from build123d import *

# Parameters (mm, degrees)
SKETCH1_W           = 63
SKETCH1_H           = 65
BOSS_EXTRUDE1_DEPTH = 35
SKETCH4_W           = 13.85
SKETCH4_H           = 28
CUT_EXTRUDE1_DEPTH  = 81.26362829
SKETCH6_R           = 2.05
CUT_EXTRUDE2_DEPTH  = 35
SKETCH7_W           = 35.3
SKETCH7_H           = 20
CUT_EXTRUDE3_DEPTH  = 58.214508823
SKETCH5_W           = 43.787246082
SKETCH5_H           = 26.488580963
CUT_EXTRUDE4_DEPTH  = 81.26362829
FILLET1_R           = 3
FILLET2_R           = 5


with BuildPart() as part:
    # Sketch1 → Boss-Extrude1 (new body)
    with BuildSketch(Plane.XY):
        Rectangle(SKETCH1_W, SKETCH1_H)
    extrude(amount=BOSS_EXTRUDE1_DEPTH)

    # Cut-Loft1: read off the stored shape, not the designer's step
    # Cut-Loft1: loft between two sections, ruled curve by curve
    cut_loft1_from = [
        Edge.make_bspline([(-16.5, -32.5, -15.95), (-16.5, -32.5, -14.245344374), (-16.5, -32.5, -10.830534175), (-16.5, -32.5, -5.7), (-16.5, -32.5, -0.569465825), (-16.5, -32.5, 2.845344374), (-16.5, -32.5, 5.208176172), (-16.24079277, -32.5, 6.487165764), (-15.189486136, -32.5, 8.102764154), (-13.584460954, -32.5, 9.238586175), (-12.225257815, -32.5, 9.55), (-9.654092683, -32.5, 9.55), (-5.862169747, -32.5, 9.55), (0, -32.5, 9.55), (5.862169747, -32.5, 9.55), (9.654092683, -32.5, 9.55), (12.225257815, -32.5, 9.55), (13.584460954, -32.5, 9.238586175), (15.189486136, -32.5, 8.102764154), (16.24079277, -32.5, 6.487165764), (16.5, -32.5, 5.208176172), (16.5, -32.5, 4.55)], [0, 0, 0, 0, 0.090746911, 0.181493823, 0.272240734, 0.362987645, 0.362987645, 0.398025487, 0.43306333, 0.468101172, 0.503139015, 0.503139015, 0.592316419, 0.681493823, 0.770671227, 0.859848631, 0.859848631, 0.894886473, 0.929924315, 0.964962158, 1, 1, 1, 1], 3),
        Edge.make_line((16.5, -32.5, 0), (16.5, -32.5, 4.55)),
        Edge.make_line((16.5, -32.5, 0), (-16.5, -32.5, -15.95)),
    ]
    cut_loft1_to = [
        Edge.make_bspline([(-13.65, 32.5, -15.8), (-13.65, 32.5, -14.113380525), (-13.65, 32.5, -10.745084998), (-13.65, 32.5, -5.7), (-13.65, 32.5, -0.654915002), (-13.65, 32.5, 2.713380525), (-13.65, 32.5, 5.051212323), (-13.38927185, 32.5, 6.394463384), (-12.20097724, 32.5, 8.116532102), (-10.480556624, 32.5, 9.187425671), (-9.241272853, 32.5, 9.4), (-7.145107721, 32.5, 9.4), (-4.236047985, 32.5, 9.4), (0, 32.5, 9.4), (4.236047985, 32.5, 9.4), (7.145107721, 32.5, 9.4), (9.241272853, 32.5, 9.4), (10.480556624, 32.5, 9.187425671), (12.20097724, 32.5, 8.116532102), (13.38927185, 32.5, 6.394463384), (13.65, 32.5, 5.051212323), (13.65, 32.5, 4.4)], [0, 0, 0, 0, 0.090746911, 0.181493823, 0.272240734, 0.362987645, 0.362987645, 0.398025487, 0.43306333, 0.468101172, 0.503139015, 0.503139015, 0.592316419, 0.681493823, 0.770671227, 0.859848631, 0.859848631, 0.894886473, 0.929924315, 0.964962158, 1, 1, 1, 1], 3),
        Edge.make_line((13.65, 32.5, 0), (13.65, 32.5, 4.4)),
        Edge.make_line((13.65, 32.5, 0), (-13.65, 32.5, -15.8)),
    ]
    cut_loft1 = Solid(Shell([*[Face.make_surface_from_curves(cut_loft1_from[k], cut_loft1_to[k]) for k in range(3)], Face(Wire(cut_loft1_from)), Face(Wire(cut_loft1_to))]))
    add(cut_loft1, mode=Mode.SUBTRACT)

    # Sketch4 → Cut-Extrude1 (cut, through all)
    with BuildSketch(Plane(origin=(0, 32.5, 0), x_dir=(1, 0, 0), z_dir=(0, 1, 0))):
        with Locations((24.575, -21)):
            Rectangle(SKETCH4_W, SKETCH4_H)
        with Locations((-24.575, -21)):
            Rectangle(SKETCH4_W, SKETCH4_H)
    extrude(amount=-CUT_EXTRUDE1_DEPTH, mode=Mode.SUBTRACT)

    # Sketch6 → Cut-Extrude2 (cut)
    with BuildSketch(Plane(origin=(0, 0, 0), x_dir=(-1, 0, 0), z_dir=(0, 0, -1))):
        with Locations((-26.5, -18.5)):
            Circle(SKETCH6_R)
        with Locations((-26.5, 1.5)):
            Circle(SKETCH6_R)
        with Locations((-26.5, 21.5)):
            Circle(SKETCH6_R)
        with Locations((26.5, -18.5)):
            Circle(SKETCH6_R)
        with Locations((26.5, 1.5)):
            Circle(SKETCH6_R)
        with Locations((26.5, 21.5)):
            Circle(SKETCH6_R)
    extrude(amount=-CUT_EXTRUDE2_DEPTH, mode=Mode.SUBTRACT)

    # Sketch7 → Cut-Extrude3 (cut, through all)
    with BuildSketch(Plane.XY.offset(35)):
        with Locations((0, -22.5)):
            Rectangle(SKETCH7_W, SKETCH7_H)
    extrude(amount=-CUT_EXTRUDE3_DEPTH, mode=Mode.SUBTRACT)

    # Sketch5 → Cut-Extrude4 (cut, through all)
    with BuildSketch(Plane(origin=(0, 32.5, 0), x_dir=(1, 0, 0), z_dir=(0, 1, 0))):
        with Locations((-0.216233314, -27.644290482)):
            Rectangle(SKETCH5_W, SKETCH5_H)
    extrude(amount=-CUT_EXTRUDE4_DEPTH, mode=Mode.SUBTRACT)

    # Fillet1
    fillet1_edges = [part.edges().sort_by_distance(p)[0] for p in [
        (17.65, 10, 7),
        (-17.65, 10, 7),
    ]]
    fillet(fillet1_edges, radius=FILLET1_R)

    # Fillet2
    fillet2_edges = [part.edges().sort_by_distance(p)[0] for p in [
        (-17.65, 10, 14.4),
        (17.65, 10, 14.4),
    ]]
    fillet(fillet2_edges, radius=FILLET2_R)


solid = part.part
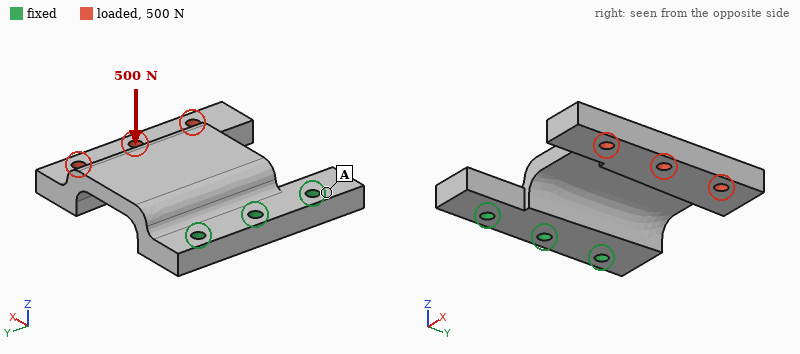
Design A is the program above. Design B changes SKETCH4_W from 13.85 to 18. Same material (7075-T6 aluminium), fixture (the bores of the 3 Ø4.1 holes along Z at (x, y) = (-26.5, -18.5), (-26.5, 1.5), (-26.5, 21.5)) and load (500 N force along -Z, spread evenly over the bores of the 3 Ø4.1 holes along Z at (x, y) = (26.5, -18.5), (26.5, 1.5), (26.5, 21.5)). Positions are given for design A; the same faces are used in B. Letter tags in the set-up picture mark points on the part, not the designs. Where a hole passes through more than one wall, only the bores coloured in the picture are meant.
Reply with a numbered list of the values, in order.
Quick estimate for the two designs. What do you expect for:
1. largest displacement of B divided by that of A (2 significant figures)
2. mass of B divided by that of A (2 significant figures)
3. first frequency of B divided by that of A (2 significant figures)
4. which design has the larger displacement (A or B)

1. 1.8
2. 0.94
3. 0.74
4. B
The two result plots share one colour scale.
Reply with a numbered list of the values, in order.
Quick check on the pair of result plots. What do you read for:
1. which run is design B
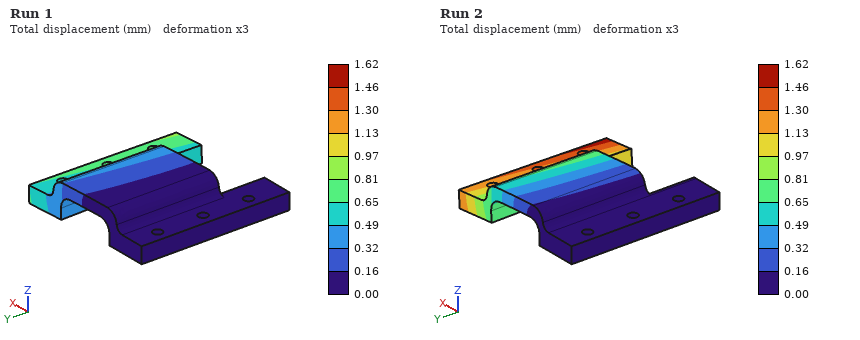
1. Run 2
